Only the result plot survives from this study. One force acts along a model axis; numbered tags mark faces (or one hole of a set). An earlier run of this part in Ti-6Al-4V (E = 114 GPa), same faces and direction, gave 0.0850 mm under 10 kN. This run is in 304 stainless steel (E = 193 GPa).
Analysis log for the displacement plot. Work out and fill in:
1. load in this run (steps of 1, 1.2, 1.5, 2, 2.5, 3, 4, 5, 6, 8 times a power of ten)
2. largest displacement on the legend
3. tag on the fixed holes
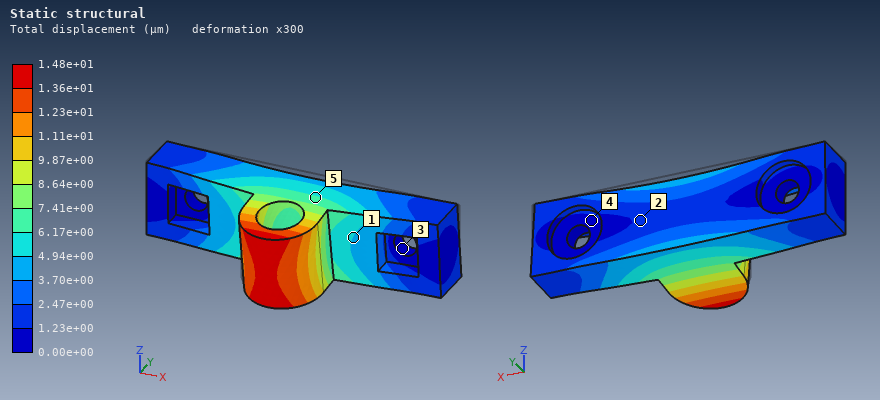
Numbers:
3 kN
1.48e+01 µm
3
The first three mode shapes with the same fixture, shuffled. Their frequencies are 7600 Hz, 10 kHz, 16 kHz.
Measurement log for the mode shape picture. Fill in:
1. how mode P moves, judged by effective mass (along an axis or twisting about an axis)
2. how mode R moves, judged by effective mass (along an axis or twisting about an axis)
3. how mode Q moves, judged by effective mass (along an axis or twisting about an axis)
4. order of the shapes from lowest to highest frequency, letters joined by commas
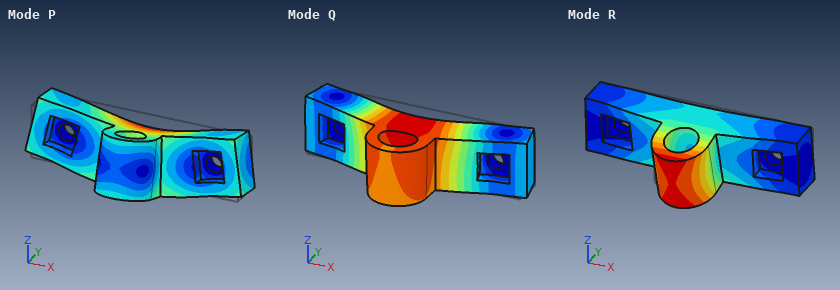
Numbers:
along Z
along Z
along Y
R, Q, P
